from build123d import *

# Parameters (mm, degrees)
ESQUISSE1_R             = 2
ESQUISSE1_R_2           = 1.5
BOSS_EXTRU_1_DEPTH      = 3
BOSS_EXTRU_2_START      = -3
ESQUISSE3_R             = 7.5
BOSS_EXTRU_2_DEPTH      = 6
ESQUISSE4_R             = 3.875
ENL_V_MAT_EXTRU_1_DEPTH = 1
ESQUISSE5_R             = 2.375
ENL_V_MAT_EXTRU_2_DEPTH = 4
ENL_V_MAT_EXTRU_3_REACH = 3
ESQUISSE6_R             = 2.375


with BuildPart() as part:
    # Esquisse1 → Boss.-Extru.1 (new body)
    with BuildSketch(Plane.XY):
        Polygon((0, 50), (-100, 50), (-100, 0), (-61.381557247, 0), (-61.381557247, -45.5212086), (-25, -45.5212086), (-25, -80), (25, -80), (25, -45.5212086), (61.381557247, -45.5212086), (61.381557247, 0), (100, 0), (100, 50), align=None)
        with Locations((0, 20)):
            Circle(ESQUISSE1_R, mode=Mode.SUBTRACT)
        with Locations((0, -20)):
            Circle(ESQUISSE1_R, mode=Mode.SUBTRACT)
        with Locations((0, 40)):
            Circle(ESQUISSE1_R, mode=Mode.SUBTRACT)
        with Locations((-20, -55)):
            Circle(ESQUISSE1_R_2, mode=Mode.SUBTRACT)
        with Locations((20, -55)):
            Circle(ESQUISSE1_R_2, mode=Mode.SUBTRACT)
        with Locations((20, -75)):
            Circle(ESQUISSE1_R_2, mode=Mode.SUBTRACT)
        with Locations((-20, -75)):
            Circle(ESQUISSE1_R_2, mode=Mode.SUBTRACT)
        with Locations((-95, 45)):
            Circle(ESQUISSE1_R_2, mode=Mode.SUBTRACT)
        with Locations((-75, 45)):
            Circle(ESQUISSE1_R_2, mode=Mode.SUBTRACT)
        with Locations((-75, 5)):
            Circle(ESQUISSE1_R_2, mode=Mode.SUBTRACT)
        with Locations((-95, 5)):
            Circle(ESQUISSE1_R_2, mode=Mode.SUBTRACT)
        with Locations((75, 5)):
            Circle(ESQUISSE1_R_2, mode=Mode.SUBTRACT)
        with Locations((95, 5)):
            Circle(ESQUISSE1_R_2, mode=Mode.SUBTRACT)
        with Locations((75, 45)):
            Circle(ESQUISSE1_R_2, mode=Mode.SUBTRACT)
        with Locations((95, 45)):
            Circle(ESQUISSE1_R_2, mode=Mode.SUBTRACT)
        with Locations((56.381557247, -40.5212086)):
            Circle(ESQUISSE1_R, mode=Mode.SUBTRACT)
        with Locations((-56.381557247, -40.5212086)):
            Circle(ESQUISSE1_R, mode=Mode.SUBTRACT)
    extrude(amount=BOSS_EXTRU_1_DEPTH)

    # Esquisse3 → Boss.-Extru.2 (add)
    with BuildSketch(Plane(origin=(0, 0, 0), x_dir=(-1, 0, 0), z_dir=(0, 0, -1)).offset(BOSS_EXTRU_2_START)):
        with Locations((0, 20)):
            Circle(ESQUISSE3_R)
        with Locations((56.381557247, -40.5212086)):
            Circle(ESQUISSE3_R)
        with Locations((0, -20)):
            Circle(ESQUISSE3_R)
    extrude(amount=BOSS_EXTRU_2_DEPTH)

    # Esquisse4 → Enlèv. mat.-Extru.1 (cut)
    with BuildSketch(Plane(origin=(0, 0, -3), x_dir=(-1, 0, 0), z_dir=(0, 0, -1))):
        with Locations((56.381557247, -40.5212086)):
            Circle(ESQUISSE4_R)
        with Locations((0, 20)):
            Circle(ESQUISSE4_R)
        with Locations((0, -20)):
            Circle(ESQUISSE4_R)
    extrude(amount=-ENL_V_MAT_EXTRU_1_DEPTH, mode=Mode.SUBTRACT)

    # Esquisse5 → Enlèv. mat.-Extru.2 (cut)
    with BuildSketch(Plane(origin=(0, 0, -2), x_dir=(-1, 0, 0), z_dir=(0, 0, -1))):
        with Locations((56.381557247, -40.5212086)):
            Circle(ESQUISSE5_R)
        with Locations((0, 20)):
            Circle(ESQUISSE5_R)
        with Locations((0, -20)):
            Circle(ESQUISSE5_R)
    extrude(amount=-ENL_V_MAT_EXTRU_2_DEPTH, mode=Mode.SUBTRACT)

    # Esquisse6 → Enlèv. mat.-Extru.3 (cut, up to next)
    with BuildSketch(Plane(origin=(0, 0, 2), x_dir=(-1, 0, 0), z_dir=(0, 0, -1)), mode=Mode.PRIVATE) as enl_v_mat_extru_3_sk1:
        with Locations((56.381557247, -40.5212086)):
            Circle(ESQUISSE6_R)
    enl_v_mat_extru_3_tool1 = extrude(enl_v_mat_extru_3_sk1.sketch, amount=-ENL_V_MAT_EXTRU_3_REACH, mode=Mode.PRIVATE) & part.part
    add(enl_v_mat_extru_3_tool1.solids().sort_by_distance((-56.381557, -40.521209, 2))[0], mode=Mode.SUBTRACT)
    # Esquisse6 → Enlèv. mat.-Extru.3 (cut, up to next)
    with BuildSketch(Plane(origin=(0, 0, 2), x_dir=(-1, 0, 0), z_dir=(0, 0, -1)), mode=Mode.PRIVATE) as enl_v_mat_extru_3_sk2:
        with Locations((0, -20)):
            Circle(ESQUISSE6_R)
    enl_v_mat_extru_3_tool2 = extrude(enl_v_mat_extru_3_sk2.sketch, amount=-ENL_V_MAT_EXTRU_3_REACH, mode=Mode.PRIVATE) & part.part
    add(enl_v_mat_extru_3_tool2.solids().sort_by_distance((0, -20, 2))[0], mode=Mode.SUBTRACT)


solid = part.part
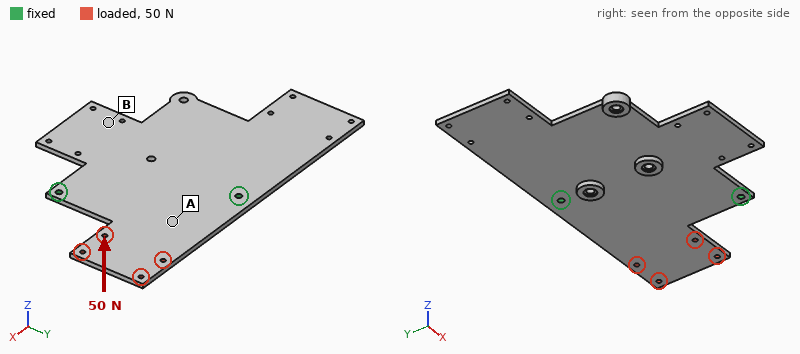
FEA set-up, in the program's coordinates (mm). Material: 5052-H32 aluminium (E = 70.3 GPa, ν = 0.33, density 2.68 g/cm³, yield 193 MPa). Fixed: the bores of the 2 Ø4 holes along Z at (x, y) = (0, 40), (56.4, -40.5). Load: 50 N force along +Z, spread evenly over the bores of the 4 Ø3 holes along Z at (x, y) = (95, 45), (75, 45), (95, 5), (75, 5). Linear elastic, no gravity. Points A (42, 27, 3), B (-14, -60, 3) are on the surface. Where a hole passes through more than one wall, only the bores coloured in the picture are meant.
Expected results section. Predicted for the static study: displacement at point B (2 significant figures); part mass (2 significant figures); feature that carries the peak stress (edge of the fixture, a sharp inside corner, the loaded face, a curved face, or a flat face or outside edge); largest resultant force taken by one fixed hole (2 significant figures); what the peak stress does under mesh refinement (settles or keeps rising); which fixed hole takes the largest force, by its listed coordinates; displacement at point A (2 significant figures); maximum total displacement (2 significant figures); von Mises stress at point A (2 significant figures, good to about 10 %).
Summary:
0.20 mm
140 g
edge of the fixture
31 N
keeps rising
(56.4, -40.5)
0.19 mm
0.95 mm
18 MPa
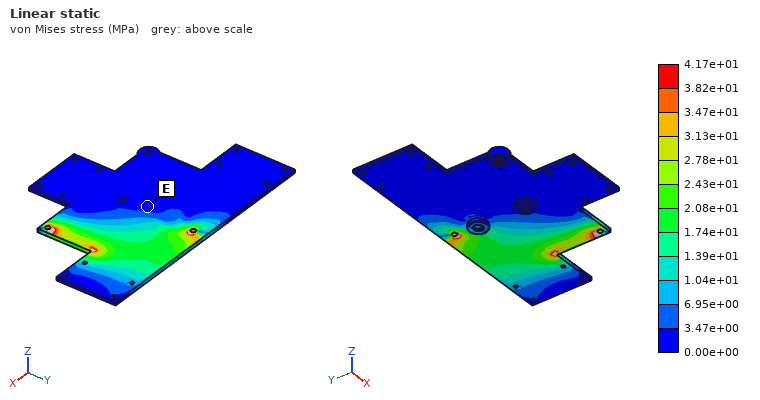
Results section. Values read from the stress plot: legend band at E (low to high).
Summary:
0.00e+00 to 3.47e+00 MPa
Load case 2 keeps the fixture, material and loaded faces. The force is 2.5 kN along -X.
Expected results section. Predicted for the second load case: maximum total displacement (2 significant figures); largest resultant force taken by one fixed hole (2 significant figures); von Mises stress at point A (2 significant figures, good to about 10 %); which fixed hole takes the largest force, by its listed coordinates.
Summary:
32 µm
1.9 kN
15 MPa
(0, 40)
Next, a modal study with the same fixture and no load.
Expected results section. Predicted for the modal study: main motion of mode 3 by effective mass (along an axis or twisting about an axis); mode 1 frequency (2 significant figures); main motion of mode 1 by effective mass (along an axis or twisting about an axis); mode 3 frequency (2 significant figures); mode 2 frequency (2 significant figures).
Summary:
along Z
220 Hz
along Z
420 Hz
360 Hz
